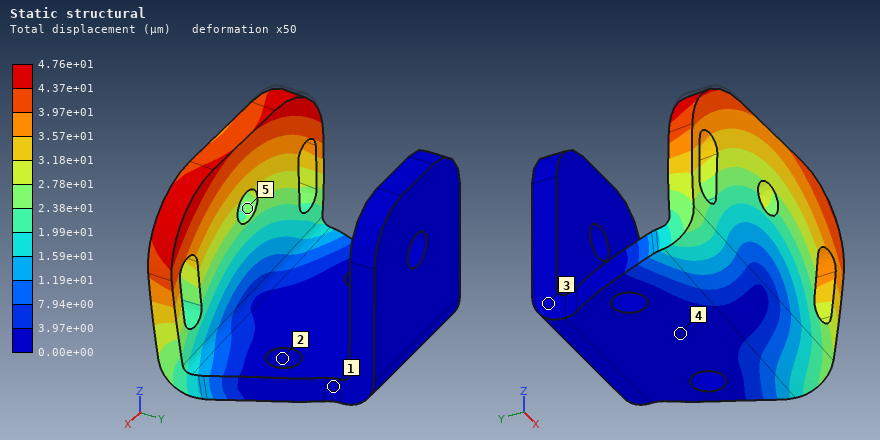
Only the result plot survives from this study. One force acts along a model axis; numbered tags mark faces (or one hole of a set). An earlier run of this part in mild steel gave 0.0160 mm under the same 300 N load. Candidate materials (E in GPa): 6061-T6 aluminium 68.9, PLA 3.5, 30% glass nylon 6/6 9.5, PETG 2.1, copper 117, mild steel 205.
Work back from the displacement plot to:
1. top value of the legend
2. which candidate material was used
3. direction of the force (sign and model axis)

4.76e+01 µm
6061-T6 aluminium
+X
